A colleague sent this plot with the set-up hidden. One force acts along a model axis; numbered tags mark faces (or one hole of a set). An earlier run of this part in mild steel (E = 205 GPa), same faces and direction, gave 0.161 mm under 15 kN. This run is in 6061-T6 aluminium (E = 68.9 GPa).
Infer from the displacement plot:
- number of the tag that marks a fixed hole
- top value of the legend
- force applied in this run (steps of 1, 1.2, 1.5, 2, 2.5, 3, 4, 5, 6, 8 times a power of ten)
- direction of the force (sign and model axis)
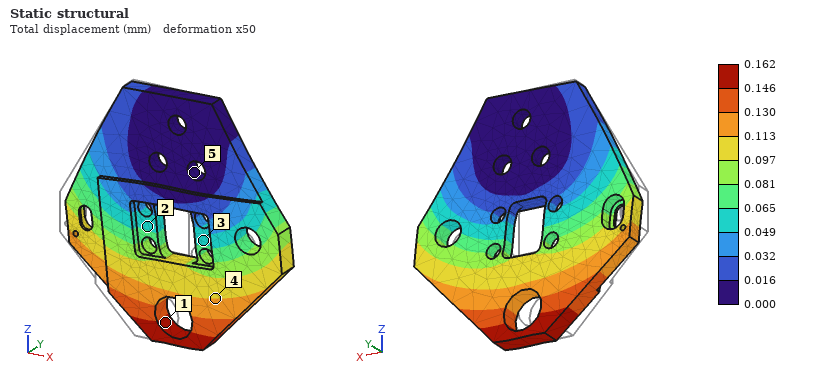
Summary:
5
0.162 mm
5 kN
+X
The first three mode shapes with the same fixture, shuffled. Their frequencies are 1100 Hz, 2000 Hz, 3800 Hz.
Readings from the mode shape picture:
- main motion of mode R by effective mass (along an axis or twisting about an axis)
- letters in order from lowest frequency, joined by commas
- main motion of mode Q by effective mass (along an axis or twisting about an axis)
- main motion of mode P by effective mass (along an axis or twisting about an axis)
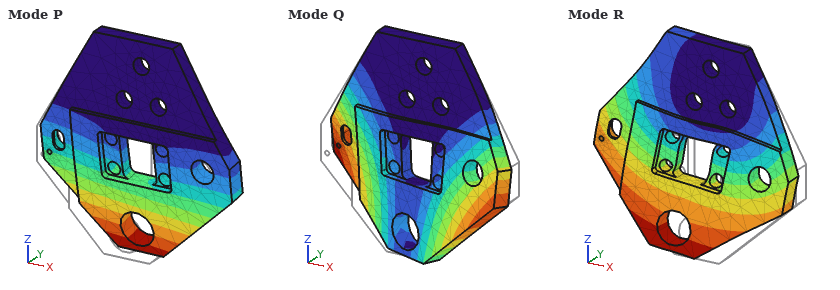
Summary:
along X
P, Q, R
twisting about Z
along Y
